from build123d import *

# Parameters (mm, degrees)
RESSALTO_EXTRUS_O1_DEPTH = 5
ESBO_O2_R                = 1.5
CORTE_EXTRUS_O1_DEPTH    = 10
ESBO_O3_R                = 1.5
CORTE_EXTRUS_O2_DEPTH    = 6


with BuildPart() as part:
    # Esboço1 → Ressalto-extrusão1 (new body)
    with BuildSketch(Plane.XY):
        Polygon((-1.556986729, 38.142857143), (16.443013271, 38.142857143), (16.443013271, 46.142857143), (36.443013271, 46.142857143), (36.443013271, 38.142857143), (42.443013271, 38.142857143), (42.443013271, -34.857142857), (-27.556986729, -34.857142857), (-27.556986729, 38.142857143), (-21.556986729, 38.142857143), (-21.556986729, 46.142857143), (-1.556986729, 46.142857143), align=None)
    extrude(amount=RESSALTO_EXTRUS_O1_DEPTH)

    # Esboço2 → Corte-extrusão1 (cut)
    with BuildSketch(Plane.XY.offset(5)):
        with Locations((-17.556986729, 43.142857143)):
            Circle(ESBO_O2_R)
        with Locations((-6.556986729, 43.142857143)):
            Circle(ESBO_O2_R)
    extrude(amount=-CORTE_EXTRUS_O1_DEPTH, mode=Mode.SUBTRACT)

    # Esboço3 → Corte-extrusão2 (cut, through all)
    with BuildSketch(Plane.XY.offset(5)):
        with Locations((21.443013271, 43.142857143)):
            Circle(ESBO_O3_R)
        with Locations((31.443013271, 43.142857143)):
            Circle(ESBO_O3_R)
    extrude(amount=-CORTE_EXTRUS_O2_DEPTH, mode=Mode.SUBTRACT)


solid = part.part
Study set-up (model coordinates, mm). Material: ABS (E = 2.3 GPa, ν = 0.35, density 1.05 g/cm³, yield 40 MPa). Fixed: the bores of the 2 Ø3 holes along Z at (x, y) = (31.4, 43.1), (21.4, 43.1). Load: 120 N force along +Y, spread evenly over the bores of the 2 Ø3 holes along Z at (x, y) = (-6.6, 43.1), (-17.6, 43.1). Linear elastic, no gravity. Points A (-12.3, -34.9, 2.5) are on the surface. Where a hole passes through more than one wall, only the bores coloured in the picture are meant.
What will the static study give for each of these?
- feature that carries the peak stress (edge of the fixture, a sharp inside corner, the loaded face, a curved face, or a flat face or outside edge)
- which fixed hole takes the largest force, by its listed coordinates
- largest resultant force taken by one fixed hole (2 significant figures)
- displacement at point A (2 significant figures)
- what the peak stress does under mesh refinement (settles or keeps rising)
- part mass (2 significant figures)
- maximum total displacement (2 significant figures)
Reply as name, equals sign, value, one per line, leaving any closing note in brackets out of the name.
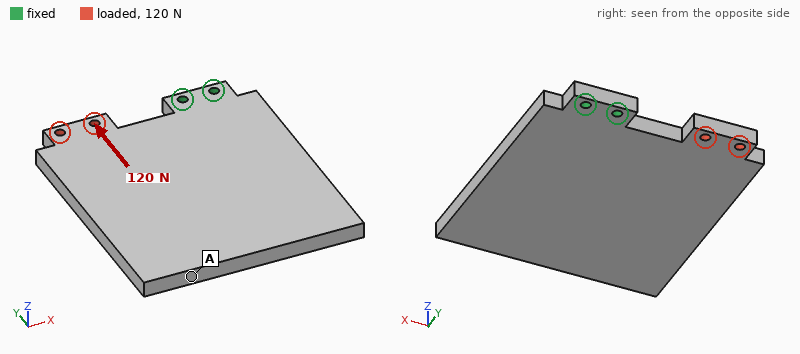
feature that carries the peak stress = edge of the fixture
which fixed hole takes the largest force, by its listed coordinates = (21.4, 43.1)
largest resultant force taken by one fixed hole = 440 N
displacement at point A = 0.80 mm
what the peak stress does under mesh refinement = keeps rising
part mass = 28 g
maximum total displacement = 0.88 mm
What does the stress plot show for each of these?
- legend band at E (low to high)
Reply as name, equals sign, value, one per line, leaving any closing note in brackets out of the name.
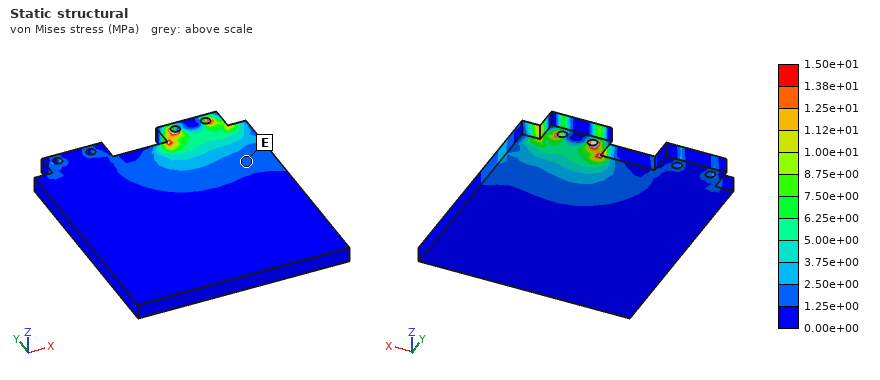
legend band at E = 1.25e+00 to 2.50e+00 MPa
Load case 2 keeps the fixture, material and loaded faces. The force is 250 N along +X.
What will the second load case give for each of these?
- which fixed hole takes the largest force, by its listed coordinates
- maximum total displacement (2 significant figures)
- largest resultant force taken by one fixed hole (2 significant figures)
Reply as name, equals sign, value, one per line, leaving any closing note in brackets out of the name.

which fixed hole takes the largest force, by its listed coordinates = (21.4, 43.1)
maximum total displacement = 0.24 mm
largest resultant force taken by one fixed hole = 140 N
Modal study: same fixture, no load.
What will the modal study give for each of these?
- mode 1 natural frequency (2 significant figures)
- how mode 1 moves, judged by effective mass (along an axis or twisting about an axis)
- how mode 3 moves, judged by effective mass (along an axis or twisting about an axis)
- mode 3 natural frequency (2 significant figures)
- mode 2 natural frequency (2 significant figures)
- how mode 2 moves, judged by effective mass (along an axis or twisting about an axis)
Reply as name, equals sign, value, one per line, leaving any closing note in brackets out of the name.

mode 1 natural frequency = 120 Hz
how mode 1 moves, judged by effective mass = along Z
how mode 3 moves, judged by effective mass = along X
mode 3 natural frequency = 410 Hz
mode 2 natural frequency = 270 Hz
how mode 2 moves, judged by effective mass = twisting about Y
